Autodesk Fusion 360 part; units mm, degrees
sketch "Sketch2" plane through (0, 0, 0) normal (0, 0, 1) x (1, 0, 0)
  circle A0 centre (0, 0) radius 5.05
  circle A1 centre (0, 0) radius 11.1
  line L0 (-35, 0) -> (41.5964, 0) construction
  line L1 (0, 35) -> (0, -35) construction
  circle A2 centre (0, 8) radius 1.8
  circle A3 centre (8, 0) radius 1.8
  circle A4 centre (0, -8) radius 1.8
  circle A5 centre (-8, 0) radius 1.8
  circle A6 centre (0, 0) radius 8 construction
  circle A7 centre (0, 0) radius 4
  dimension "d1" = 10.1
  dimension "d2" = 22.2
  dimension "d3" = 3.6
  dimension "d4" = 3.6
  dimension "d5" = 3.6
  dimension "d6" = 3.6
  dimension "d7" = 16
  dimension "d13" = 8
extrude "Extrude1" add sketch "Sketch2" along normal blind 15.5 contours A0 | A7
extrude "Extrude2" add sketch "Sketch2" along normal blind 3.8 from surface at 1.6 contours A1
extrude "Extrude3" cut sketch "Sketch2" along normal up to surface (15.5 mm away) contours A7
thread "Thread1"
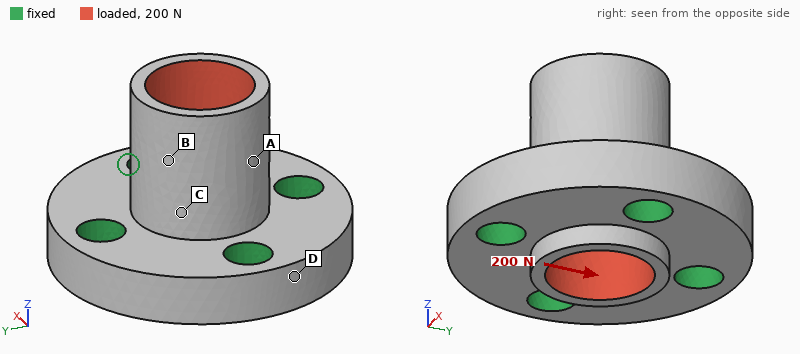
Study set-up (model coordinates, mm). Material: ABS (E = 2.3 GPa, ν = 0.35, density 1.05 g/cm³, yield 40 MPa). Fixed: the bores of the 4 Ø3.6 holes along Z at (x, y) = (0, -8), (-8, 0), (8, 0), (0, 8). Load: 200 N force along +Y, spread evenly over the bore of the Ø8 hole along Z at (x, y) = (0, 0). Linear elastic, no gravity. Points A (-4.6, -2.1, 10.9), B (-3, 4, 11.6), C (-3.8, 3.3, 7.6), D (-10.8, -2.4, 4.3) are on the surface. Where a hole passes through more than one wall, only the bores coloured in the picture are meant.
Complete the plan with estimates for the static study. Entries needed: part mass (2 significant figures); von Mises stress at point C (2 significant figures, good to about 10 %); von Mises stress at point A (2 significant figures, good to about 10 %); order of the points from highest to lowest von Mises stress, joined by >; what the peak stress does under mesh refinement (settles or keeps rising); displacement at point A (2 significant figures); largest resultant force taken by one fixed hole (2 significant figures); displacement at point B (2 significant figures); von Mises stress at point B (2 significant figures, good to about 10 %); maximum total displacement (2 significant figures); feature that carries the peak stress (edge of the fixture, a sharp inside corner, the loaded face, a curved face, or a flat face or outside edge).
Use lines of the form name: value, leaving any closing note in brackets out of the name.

part mass: 1.5 g
von Mises stress at point C: 7.6 MPa
von Mises stress at point A: 6.0 MPa
order of the points from highest to lowest von Mises stress, joined by >: C > A > B > D
what the peak stress does under mesh refinement: keeps rising
displacement at point A: 0.065 mm
largest resultant force taken by one fixed hole: 84 N
displacement at point B: 0.076 mm
von Mises stress at point B: 3.9 MPa
maximum total displacement: 0.11 mm
feature that carries the peak stress: a sharp inside corner
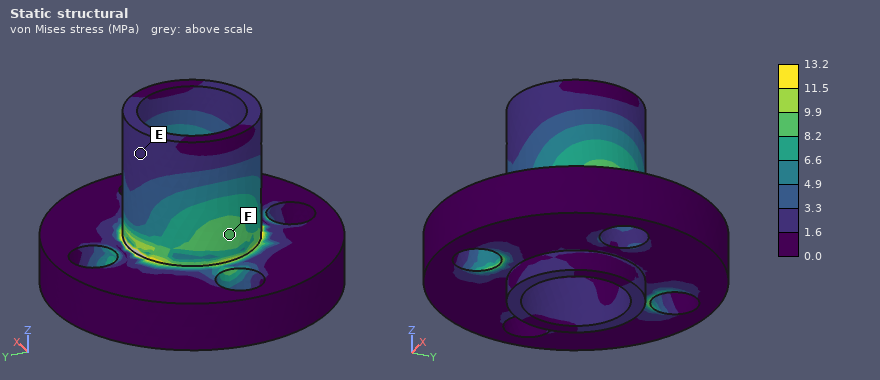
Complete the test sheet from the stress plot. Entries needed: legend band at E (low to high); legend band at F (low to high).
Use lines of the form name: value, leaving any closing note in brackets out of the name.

legend band at E: 1.6 to 3.3 MPa
legend band at F: 8.2 to 9.9 MPa
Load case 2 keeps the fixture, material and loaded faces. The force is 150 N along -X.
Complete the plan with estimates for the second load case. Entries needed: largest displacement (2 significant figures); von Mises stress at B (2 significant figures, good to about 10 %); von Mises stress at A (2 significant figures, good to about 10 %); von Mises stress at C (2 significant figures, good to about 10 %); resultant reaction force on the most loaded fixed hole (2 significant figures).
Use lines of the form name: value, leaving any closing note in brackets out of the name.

largest displacement: 80 µm
von Mises stress at B: 3.5 MPa
von Mises stress at A: 2.8 MPa
von Mises stress at C: 5.4 MPa
resultant reaction force on the most loaded fixed hole: 63 N
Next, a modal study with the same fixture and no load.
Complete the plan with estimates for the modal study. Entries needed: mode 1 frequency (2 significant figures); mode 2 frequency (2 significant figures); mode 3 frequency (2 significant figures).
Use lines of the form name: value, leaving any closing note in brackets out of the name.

mode 1 frequency: 12 kHz
mode 2 frequency: 12 kHz
mode 3 frequency: 12 kHz
